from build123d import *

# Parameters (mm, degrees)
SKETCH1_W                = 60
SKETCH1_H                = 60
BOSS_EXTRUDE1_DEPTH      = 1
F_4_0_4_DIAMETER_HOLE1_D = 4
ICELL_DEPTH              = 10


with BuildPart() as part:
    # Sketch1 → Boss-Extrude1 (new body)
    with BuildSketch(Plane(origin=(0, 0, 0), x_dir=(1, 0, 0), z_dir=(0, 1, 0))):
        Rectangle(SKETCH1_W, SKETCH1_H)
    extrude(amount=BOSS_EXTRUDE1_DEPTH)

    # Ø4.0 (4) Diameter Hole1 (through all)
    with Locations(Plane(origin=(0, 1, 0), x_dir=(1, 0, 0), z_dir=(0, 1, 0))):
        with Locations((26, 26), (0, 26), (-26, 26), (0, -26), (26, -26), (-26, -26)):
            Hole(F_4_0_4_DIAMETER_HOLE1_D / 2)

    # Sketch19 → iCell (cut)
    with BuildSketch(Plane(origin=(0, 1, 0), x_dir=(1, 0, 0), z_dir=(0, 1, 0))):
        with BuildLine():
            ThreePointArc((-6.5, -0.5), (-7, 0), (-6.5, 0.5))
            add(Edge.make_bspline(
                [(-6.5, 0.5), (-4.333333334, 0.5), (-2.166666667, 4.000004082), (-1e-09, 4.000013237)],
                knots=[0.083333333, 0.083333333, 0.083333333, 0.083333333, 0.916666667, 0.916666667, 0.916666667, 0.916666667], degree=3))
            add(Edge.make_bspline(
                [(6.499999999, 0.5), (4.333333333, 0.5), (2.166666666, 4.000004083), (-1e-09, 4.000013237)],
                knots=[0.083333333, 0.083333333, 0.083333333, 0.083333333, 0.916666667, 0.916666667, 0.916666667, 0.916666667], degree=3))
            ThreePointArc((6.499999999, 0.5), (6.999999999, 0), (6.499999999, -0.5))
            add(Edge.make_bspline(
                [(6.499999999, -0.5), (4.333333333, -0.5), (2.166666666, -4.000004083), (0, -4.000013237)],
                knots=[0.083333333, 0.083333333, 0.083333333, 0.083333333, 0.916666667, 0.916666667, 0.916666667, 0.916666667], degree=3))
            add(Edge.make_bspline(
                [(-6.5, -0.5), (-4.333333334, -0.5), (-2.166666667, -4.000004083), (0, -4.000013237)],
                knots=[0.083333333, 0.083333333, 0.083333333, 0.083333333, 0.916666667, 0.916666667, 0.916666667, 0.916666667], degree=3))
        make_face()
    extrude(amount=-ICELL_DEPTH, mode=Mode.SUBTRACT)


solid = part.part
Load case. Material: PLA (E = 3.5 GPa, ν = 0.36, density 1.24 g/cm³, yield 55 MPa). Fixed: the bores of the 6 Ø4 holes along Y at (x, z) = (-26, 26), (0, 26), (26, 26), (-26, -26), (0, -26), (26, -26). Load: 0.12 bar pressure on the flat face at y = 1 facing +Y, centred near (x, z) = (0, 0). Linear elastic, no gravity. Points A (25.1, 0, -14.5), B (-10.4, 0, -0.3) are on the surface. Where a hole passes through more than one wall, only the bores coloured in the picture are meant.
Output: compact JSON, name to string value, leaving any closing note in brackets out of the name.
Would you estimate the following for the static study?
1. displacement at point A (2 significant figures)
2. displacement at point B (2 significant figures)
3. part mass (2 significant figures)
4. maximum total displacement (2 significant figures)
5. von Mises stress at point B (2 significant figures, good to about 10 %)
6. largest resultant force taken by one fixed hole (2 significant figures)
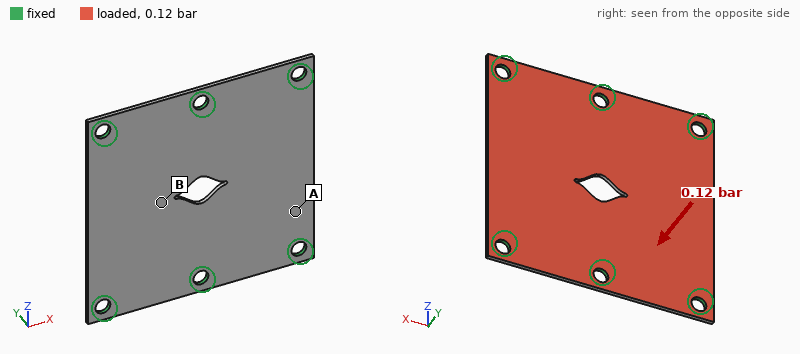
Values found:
{"displacement at point A": "0.32 mm", "displacement at point B": "0.78 mm", "part mass": "4.3 g", "maximum total displacement": "0.84 mm", "von Mises stress at point B": "9.7 MPa", "largest resultant force taken by one fixed hole": "9.2 N"}
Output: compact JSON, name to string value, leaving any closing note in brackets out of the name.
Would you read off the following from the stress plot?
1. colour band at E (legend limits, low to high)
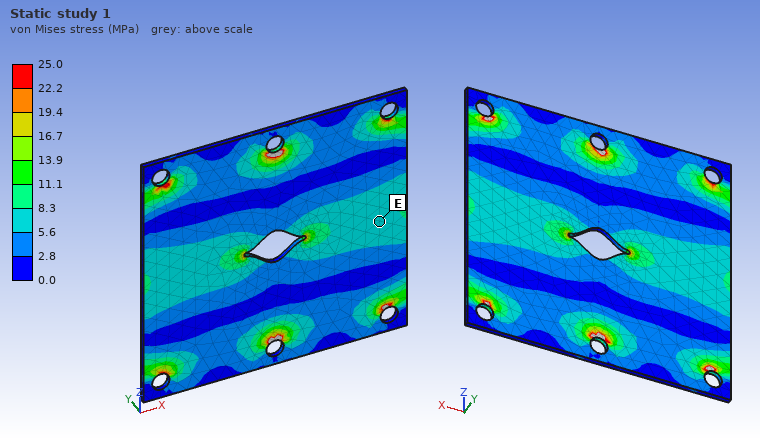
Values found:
{"colour band at E": "5.6 to 8.3 MPa"}
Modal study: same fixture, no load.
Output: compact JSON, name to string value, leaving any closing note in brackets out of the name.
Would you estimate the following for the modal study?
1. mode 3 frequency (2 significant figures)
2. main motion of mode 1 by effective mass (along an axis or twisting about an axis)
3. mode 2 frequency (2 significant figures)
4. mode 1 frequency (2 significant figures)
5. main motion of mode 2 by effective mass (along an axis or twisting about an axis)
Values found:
{"mode 3 frequency": "1200 Hz", "main motion of mode 1 by effective mass": "along Y", "mode 2 frequency": "780 Hz", "mode 1 frequency": "650 Hz", "main motion of mode 2 by effective mass": "twisting about Z"}
